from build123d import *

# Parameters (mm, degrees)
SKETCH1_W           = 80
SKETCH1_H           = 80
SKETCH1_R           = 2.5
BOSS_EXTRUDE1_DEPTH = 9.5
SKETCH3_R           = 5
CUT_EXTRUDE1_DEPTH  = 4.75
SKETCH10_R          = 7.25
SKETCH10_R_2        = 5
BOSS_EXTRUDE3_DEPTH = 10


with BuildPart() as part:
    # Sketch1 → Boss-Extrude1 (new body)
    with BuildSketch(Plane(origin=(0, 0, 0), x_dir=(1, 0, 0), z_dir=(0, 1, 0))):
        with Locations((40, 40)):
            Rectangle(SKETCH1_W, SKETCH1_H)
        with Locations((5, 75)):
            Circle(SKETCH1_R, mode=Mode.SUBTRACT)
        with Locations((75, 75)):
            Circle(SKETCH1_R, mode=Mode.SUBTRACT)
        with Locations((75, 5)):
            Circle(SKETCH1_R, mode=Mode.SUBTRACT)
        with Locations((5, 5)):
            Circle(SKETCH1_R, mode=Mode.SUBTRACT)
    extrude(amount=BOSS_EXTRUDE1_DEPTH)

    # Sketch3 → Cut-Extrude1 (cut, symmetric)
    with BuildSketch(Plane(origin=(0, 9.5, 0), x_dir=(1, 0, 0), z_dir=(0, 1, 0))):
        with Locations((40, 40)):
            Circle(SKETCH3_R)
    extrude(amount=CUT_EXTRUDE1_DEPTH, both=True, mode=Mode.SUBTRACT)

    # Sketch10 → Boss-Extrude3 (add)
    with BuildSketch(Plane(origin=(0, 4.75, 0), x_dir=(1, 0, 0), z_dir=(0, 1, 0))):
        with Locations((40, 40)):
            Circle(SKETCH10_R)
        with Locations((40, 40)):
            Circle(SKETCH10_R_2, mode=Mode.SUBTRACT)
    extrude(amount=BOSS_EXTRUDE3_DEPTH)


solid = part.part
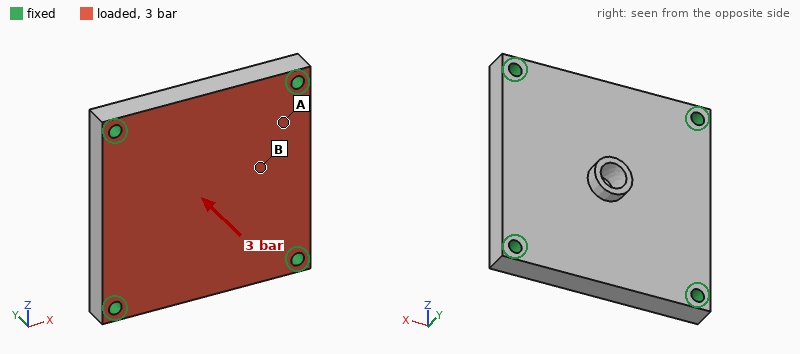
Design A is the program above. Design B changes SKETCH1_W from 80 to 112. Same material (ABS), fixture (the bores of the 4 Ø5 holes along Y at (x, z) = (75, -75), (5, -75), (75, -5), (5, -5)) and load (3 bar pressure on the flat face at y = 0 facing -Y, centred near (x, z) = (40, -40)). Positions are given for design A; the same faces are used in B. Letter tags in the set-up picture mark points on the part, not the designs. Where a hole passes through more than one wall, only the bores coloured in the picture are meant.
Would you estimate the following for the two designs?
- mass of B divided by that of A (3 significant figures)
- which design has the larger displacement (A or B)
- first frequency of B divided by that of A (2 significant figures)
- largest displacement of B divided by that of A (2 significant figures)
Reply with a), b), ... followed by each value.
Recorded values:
a) 1.40
b) A
c) 1.0
d) 0.92
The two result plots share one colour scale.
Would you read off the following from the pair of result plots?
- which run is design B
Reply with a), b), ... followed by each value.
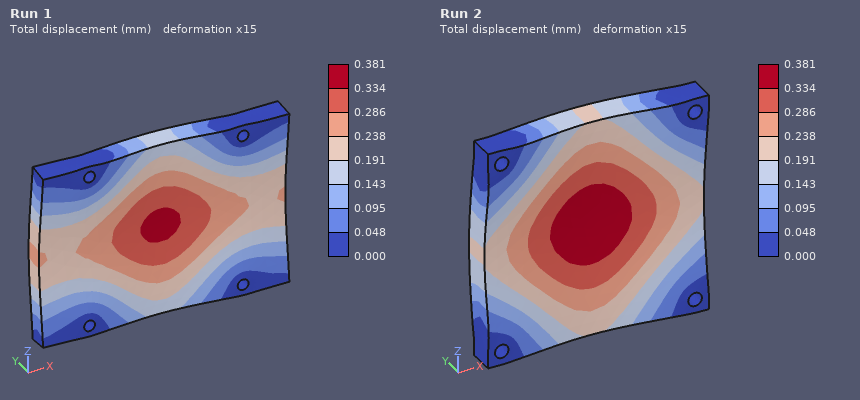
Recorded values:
a) Run 1
